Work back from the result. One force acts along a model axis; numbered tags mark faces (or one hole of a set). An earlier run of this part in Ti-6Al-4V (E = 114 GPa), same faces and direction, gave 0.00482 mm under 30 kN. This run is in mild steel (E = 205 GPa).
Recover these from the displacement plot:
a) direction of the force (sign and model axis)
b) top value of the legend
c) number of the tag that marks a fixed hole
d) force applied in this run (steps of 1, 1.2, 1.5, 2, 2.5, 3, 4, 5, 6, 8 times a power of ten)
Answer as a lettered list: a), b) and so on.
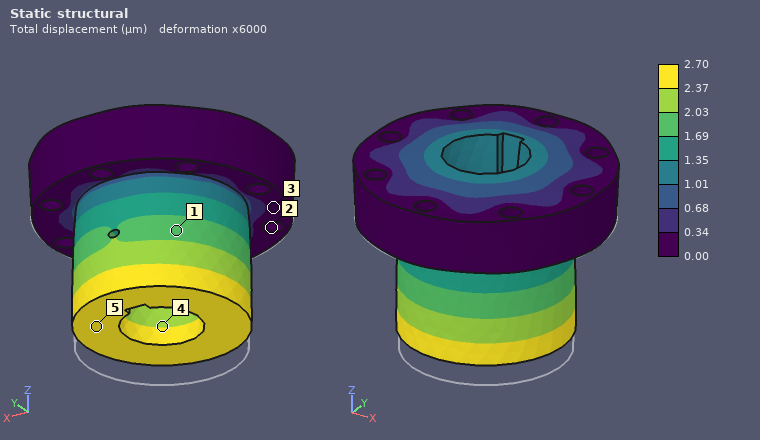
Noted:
a) +Z
b) 2.70 µm
c) 2
d) 30 kN
